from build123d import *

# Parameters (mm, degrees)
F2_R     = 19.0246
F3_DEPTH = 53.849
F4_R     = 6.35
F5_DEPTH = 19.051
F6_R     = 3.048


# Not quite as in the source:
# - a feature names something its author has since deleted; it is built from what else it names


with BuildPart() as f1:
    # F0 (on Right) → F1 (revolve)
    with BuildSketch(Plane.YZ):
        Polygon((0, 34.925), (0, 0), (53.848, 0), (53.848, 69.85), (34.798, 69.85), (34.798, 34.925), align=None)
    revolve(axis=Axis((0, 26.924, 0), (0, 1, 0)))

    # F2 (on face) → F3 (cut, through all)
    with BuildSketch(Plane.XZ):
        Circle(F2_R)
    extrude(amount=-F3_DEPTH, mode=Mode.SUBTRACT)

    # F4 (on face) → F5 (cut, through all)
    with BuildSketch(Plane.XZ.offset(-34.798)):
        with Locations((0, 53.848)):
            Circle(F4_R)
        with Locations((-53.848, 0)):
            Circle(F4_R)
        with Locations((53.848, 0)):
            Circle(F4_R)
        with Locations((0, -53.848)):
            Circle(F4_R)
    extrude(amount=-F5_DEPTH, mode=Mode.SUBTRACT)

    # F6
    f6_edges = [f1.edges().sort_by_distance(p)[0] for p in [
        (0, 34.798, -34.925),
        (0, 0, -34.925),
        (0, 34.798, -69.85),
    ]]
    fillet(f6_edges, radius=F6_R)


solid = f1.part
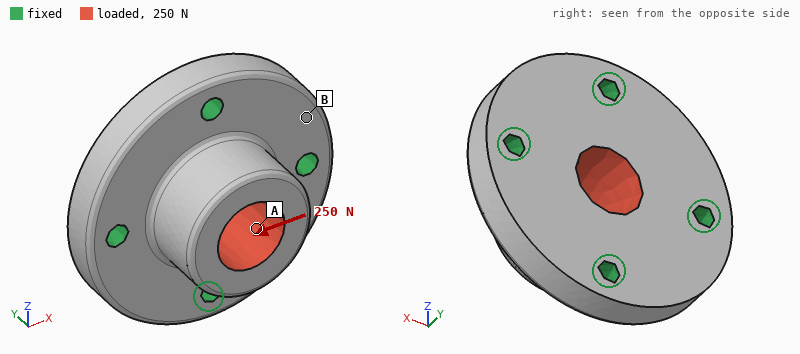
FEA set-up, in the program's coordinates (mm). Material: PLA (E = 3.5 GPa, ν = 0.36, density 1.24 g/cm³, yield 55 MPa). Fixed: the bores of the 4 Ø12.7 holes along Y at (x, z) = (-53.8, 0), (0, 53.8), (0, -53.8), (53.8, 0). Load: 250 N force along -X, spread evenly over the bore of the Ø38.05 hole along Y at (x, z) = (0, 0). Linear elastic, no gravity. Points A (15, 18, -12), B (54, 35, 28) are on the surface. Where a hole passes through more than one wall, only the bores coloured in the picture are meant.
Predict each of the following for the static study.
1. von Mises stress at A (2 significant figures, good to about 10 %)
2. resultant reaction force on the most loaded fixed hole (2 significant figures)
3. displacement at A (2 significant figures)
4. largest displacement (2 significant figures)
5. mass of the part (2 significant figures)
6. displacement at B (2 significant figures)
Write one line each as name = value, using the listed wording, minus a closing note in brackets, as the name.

von Mises stress at A = 0.10 MPa
resultant reaction force on the most loaded fixed hole = 90 N
displacement at A = 2.7 µm
largest displacement = 4.1 µm
mass of the part = 440 g
displacement at B = 0.76 µm
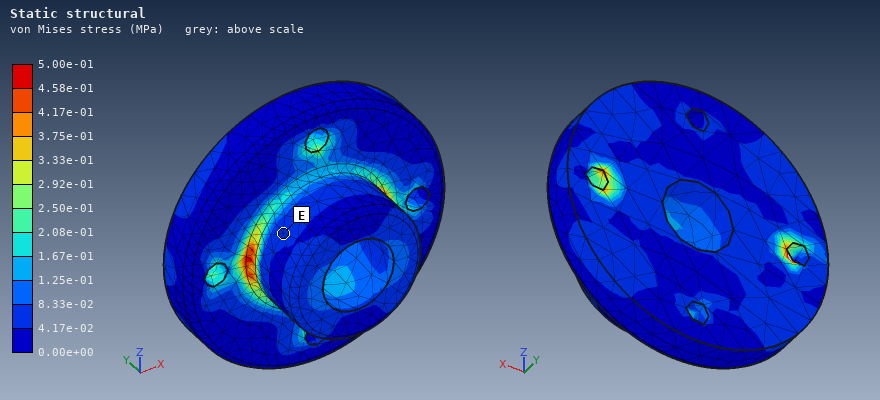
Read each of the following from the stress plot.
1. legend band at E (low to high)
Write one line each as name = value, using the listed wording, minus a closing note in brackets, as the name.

legend band at E = 4.17e-02 to 8.33e-02 MPa
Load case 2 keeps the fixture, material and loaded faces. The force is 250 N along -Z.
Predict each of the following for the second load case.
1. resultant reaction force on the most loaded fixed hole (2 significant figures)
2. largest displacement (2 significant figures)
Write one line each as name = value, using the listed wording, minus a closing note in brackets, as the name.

resultant reaction force on the most loaded fixed hole = 90 N
largest displacement = 4.1 µm
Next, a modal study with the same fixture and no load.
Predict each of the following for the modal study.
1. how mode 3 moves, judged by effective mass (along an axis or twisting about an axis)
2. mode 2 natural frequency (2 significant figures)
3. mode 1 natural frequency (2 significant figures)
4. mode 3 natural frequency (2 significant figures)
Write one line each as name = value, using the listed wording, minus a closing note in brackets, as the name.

how mode 3 moves, judged by effective mass = along Y
mode 2 natural frequency = 3100 Hz
mode 1 natural frequency = 3100 Hz
mode 3 natural frequency = 3200 Hz
